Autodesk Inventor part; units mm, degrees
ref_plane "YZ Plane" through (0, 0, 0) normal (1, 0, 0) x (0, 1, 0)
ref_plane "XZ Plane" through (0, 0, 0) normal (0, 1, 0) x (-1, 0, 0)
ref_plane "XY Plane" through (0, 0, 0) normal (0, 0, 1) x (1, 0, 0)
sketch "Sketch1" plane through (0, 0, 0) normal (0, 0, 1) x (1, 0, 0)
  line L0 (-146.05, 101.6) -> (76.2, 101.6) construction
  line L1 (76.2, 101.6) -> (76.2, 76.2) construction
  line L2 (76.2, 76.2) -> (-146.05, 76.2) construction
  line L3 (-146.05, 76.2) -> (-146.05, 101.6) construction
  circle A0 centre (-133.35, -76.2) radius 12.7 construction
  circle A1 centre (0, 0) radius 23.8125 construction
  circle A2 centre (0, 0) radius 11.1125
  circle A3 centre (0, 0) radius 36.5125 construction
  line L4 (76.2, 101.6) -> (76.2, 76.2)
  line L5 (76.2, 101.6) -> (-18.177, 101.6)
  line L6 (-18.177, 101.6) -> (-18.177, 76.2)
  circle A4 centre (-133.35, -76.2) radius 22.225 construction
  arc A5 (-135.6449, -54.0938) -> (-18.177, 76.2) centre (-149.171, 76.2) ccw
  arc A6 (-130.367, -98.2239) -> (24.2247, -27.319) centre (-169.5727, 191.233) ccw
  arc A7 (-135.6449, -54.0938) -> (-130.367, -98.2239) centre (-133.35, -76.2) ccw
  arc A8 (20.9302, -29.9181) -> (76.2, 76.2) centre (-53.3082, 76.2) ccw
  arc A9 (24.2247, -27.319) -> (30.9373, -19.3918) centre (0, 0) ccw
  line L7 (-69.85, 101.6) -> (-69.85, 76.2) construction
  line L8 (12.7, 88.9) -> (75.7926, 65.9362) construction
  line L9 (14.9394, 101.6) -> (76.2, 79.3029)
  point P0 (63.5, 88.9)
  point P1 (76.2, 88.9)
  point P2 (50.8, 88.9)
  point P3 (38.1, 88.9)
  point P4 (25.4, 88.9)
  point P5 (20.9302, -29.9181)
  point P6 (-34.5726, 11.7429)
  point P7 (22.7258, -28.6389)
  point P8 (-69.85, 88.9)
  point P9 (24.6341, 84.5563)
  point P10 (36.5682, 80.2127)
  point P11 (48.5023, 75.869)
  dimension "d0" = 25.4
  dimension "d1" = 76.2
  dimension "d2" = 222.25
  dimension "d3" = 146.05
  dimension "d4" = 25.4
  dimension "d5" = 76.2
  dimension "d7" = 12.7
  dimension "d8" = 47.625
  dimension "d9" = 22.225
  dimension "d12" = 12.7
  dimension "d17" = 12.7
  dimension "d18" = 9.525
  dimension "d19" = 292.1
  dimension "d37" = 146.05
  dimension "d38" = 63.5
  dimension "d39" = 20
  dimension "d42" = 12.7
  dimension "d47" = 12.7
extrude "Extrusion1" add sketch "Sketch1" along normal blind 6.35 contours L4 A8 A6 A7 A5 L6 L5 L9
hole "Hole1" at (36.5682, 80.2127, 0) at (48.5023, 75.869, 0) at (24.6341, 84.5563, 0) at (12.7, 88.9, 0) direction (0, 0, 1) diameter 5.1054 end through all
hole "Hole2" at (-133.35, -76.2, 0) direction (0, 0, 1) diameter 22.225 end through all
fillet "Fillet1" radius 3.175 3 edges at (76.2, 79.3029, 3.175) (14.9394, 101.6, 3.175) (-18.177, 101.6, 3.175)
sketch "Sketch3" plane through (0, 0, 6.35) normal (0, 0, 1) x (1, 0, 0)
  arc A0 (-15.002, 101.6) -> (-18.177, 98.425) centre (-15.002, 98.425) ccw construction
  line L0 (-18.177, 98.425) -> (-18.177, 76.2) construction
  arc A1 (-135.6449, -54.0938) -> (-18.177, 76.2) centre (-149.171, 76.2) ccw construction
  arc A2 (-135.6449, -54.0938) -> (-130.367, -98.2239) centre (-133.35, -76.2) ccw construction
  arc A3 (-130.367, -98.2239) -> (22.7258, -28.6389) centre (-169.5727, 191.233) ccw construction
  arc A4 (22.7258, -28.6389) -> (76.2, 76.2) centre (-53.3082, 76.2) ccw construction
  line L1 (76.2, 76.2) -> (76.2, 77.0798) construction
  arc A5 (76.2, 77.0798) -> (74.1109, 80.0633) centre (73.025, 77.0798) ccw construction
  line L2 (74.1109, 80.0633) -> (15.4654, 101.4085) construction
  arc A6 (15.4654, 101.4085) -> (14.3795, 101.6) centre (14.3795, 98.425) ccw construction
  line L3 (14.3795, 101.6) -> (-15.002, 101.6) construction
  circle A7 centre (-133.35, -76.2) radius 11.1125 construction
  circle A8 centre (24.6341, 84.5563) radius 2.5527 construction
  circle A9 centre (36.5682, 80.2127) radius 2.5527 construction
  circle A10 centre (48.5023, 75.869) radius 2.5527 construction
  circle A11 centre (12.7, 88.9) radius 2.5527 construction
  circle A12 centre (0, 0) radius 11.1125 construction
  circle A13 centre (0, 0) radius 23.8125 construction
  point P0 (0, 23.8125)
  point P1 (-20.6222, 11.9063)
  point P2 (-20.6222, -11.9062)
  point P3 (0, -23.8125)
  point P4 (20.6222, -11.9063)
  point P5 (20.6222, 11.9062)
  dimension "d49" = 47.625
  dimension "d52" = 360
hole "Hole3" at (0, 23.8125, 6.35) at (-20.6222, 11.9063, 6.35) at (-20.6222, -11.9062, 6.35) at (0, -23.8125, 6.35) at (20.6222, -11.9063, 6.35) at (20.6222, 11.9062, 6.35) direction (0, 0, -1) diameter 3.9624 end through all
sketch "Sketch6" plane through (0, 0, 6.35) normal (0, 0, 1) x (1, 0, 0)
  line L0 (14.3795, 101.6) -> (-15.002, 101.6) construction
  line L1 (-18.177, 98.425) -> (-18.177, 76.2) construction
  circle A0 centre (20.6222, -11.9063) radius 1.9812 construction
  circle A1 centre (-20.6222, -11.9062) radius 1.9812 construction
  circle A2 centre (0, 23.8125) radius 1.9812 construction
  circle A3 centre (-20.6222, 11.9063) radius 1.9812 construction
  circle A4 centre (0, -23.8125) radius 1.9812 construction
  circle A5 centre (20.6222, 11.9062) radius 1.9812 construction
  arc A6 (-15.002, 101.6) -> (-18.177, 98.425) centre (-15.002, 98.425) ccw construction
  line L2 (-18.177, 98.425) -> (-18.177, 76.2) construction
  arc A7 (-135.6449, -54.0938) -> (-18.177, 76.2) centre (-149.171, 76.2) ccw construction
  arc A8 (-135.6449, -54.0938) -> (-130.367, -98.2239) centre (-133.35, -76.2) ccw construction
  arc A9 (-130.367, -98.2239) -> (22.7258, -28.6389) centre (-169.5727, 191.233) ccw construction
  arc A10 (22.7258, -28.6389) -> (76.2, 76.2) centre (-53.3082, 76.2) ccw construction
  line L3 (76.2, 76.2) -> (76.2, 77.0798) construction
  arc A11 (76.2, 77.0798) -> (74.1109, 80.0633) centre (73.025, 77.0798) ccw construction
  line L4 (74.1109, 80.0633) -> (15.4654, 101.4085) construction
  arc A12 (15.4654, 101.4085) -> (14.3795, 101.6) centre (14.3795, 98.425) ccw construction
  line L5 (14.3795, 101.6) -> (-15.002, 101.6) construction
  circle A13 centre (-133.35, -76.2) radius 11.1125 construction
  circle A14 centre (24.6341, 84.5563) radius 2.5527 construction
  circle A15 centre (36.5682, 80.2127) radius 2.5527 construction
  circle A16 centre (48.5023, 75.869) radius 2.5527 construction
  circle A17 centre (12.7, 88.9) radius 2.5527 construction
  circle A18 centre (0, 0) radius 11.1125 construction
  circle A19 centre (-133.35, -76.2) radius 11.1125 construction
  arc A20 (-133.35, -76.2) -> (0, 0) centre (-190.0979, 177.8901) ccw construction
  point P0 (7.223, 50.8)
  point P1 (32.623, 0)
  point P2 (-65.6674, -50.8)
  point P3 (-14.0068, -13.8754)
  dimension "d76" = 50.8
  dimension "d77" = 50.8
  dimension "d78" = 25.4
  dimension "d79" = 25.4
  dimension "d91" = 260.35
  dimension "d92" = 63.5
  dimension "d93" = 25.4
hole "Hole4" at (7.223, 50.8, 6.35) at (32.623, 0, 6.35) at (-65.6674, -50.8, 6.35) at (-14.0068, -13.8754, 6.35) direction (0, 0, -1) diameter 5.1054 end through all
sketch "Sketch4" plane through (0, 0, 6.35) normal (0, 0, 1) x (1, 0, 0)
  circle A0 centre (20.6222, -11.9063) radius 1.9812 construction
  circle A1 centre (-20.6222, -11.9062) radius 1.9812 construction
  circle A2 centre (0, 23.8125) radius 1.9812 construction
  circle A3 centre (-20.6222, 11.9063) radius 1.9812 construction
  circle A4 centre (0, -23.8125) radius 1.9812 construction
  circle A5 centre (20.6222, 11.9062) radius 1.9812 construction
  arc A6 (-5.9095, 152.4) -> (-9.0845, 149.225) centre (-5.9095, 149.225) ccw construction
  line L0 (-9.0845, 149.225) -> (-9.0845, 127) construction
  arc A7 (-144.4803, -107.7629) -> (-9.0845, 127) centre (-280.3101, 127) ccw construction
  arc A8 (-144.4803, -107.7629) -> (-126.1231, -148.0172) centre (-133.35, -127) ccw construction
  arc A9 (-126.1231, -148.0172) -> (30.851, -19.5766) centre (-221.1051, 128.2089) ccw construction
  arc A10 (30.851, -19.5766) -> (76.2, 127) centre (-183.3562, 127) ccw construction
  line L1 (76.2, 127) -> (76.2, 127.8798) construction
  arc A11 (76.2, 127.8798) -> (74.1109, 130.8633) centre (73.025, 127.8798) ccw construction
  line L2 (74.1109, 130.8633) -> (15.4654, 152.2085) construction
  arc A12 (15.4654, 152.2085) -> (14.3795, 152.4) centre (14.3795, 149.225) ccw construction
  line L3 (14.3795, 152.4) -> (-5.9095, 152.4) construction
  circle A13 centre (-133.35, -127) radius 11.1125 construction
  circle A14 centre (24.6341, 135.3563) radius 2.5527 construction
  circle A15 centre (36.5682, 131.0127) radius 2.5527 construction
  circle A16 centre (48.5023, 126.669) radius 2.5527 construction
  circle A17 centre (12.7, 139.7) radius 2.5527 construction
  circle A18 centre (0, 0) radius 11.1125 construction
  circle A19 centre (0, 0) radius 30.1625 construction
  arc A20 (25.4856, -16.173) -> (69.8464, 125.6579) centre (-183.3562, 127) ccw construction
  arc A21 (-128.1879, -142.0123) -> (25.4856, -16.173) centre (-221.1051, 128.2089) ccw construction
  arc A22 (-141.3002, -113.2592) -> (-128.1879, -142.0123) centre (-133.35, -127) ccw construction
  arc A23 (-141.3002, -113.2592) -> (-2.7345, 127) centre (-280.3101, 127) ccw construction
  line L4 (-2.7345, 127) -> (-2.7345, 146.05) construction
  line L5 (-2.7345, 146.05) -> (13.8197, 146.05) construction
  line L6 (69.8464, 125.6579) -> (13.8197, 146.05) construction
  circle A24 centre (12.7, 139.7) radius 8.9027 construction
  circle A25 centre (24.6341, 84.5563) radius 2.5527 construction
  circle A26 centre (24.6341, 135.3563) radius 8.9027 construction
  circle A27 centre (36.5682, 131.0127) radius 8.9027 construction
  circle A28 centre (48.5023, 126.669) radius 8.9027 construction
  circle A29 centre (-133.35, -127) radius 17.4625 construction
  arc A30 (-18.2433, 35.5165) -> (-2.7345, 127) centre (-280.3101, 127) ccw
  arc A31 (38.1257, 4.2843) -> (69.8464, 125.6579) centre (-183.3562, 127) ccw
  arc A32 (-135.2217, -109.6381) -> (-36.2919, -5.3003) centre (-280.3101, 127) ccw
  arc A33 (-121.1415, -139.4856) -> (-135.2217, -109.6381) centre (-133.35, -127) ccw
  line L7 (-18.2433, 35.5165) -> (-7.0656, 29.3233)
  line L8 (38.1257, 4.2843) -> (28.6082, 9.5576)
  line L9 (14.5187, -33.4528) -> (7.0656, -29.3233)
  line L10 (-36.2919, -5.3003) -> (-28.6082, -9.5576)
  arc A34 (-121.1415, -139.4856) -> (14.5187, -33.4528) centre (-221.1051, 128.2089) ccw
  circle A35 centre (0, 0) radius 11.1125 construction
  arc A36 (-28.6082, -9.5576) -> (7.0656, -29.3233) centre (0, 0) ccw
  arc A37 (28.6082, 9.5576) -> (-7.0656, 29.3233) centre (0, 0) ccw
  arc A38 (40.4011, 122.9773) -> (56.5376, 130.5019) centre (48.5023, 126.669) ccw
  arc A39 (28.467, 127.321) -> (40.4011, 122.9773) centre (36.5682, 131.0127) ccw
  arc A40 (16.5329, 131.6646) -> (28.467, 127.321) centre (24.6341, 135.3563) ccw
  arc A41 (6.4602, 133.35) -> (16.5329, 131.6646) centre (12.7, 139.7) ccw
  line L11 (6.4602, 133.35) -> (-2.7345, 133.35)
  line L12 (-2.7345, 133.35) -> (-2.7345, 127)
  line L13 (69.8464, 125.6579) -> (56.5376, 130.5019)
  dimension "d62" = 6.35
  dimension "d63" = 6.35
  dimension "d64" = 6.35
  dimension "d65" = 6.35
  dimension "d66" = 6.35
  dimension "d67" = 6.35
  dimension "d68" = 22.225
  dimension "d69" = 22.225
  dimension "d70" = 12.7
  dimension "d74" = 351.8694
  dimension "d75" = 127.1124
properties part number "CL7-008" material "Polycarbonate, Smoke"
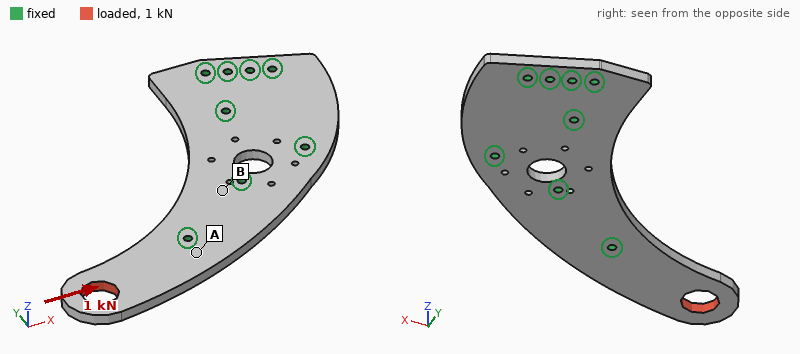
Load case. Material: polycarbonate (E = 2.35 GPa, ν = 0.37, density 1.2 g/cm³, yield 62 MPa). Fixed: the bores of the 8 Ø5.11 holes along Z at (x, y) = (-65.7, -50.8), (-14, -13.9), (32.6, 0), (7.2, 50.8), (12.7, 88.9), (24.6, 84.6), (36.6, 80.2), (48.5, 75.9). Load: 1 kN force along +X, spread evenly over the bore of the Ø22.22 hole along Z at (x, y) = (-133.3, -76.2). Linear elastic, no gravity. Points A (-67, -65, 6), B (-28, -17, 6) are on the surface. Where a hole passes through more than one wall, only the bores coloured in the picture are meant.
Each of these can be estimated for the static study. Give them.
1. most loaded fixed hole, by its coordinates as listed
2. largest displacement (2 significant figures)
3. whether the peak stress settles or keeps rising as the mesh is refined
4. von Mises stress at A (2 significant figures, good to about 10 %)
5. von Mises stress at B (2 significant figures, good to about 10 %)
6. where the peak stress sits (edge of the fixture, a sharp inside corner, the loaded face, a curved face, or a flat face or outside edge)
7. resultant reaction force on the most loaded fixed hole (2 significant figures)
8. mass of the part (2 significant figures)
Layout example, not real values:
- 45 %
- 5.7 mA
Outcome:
- (-65.7, -50.8)
- 1.0 mm
- keeps rising
- 5.8 MPa
- 1.7 MPa
- edge of the fixture
- 1.0 kN
- 130 g
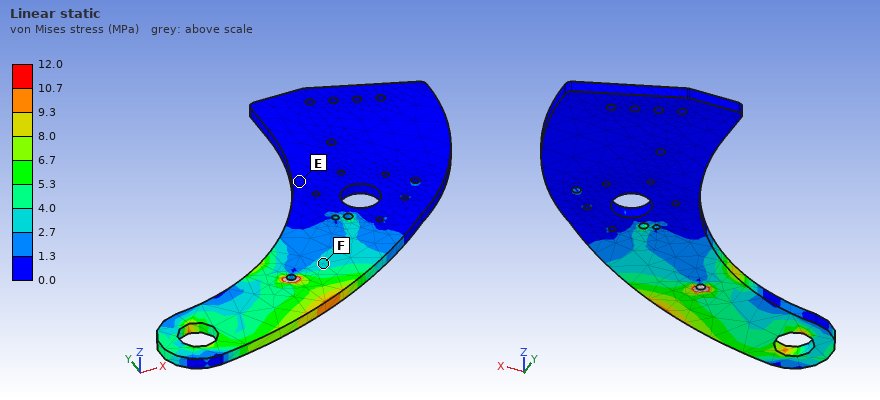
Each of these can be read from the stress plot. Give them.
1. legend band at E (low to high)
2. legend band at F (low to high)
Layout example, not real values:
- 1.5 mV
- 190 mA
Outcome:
- 0.0 to 1.3 MPa
- 2.7 to 4.0 MPa
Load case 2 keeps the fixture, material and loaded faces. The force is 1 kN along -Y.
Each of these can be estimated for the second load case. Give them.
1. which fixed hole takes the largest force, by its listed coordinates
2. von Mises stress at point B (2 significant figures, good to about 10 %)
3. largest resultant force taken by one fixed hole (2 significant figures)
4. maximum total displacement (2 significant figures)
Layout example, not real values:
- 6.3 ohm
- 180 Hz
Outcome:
- (-65.7, -50.8)
- 6.2 MPa
- 1.9 kN
- 3.1 mm
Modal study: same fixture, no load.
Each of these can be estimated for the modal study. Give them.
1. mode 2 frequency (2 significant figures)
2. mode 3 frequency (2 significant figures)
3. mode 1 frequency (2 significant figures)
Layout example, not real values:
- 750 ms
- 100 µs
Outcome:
- 640 Hz
- 910 Hz
- 190 Hz
